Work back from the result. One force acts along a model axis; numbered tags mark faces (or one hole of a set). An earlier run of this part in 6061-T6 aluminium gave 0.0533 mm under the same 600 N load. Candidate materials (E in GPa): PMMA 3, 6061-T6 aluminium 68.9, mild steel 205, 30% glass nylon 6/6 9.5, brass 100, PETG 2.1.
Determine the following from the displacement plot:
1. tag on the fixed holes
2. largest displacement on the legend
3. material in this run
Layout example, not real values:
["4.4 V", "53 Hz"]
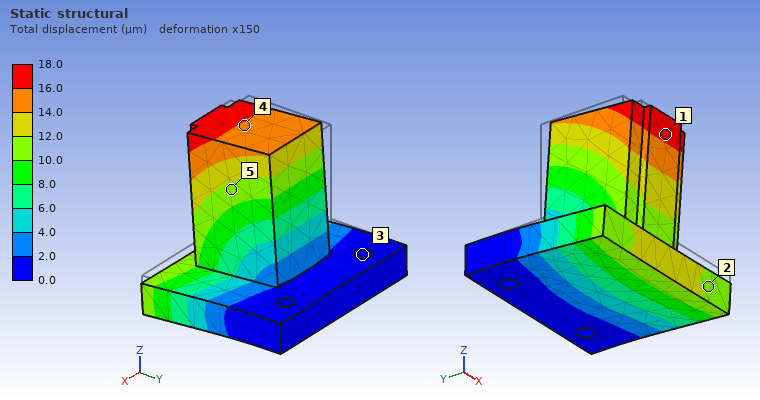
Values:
["3", "18.0 µm", "mild steel"]
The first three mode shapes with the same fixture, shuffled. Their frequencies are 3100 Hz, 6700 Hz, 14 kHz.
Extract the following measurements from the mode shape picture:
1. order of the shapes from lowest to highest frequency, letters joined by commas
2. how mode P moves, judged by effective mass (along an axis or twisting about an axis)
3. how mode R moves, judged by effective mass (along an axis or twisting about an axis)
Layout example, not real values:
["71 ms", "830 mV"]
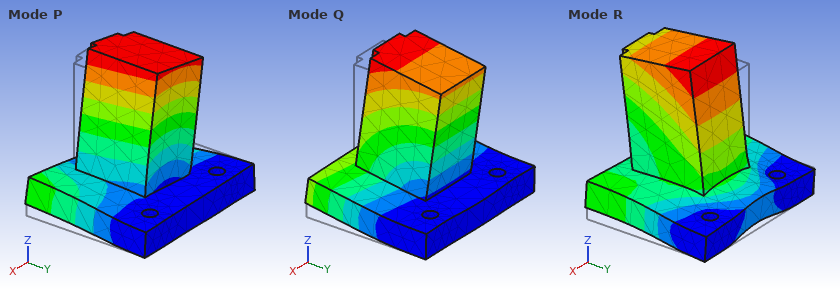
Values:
["Q, P, R", "along X", "along Z"]
